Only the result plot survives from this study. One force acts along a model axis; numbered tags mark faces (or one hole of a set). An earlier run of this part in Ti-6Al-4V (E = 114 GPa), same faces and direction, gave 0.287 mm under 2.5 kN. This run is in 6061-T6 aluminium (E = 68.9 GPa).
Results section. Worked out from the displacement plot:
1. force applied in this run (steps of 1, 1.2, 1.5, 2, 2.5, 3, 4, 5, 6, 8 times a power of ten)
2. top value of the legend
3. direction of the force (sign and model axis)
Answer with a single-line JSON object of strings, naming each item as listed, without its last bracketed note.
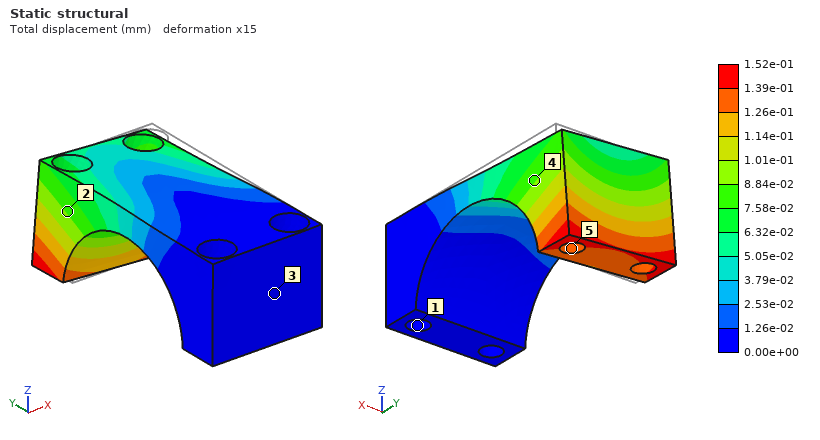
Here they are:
{"force applied in this run": "800 N", "top value of the legend": "1.52e-01 mm", "direction of the force": "-X"}
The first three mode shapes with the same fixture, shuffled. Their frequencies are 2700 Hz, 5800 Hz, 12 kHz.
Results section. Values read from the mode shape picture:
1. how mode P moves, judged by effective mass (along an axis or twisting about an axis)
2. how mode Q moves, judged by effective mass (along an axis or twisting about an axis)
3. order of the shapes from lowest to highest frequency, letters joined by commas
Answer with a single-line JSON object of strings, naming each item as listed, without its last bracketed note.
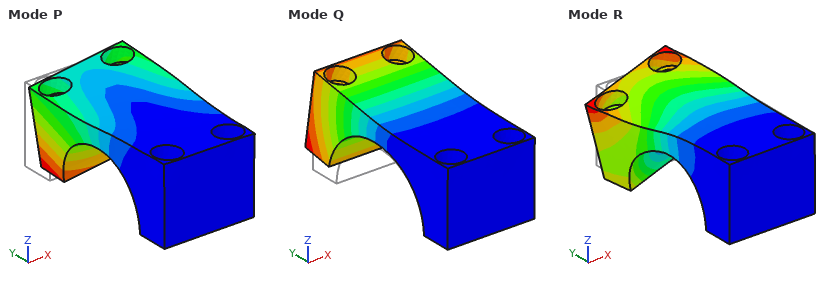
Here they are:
{"how mode P moves, judged by effective mass": "along X", "how mode Q moves, judged by effective mass": "along Z", "order of the shapes from lowest to highest frequency, letters joined by commas": "Q, P, R"}
